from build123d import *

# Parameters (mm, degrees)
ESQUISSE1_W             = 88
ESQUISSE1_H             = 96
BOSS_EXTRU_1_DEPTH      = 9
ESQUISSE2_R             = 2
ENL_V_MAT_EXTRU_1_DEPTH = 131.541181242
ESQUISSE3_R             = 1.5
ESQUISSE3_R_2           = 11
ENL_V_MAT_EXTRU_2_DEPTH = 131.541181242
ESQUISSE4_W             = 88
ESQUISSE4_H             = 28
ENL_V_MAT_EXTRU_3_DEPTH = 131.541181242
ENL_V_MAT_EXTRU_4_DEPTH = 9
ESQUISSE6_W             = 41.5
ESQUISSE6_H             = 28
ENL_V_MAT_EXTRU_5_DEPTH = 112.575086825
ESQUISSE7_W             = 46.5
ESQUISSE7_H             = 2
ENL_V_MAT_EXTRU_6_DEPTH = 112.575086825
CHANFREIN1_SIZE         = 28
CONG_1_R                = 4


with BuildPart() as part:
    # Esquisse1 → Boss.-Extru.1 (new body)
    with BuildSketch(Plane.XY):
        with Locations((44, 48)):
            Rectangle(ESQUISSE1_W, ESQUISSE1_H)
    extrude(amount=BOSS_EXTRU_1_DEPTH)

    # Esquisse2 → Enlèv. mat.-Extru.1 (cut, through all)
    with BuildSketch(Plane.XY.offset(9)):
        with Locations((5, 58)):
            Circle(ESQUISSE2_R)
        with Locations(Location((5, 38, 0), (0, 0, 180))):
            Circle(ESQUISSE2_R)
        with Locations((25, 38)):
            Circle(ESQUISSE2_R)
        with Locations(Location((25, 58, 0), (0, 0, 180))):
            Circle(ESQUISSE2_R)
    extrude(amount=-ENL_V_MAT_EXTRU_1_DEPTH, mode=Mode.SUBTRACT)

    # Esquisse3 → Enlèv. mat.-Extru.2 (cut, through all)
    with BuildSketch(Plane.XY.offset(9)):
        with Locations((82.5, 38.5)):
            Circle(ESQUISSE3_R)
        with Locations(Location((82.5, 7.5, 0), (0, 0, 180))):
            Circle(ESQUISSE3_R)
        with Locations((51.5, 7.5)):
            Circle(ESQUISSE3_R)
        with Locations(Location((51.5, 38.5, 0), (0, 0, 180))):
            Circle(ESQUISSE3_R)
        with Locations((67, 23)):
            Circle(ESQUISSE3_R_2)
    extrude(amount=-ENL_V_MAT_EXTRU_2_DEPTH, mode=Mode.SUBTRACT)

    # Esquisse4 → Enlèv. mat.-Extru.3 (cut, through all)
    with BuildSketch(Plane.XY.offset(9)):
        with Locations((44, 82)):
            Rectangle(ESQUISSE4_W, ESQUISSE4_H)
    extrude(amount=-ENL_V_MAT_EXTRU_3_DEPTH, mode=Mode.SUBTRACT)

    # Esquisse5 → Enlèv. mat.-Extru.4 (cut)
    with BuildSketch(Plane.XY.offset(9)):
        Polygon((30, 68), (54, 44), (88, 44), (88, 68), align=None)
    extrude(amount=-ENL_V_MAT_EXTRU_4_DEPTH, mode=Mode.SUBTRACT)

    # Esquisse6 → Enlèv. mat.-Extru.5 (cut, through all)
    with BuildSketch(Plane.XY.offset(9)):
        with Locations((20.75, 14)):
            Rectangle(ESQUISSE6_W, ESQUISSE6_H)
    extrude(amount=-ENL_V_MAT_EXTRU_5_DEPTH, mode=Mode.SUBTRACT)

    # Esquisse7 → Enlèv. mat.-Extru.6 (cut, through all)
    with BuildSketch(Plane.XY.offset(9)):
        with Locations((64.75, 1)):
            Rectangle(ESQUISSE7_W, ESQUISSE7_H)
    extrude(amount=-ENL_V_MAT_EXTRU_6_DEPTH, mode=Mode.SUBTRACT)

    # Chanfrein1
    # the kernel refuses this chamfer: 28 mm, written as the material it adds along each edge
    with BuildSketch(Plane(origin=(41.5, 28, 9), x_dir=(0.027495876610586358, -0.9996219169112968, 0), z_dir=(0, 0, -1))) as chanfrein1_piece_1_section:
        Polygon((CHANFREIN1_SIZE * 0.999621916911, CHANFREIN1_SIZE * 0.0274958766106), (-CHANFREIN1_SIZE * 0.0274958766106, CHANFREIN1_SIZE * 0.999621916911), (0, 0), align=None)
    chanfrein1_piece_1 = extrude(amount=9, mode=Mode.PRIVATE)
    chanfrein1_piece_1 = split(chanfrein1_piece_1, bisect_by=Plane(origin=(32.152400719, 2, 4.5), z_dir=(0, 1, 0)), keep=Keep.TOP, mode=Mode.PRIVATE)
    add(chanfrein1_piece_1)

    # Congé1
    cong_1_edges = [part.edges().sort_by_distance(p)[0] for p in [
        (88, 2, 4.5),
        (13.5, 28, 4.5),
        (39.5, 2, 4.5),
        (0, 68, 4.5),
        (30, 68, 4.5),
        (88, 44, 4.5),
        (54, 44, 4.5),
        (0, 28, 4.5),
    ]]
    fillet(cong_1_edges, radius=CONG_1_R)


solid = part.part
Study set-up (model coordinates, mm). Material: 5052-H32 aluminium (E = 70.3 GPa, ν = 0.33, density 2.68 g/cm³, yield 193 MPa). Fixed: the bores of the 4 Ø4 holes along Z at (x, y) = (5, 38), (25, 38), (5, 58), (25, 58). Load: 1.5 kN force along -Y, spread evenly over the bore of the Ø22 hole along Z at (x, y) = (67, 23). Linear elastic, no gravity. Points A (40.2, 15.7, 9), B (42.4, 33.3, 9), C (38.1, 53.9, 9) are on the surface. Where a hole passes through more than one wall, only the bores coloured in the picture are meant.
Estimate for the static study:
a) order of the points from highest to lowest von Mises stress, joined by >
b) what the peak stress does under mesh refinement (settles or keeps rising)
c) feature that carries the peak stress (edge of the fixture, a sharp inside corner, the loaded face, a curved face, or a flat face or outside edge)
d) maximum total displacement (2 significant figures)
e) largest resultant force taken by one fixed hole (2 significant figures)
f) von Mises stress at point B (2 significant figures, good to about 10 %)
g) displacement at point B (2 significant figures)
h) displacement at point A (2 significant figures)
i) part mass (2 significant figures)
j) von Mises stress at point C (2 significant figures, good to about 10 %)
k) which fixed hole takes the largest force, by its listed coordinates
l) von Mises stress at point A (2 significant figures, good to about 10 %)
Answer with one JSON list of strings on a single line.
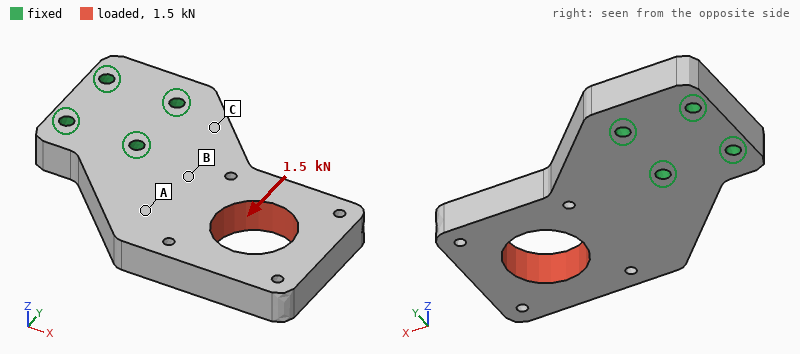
["C > B > A", "keeps rising", "edge of the fixture", "56 µm", "2.2 kN", "12 MPa", "9.4 µm", "16 µm", "85 g", "20 MPa", "(25, 58)", "5.4 MPa"]
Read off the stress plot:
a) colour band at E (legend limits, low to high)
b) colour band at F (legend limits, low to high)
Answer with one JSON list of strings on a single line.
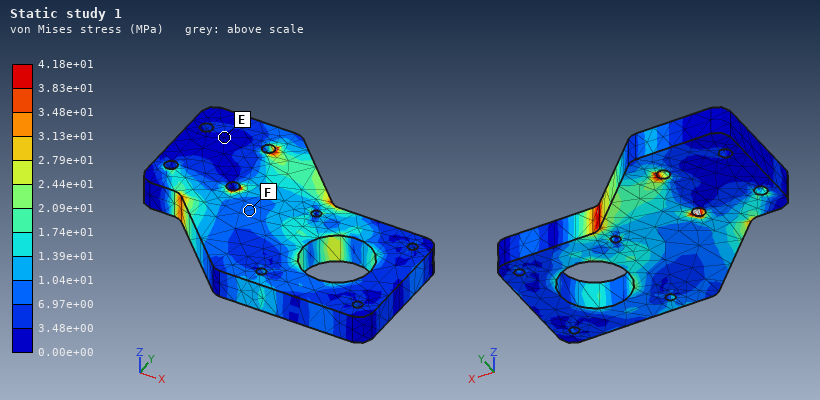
["0.00e+00 to 3.48e+00 MPa", "6.97e+00 to 1.04e+01 MPa"]
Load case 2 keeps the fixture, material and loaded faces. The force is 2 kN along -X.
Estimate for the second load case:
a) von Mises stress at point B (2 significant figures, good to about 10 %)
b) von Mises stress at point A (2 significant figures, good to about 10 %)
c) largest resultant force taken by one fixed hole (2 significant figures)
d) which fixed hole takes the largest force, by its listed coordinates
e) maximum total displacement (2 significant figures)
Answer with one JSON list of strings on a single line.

["10 MPa", "7.5 MPa", "1.8 kN", "(25, 38)", "28 µm"]
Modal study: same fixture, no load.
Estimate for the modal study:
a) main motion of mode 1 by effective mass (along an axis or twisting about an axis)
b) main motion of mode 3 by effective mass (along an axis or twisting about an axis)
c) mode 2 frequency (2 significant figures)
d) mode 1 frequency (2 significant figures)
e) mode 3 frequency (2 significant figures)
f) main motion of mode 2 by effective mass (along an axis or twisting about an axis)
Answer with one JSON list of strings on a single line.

["along Z", "along Y", "4200 Hz", "1700 Hz", "4900 Hz", "twisting about X"]
